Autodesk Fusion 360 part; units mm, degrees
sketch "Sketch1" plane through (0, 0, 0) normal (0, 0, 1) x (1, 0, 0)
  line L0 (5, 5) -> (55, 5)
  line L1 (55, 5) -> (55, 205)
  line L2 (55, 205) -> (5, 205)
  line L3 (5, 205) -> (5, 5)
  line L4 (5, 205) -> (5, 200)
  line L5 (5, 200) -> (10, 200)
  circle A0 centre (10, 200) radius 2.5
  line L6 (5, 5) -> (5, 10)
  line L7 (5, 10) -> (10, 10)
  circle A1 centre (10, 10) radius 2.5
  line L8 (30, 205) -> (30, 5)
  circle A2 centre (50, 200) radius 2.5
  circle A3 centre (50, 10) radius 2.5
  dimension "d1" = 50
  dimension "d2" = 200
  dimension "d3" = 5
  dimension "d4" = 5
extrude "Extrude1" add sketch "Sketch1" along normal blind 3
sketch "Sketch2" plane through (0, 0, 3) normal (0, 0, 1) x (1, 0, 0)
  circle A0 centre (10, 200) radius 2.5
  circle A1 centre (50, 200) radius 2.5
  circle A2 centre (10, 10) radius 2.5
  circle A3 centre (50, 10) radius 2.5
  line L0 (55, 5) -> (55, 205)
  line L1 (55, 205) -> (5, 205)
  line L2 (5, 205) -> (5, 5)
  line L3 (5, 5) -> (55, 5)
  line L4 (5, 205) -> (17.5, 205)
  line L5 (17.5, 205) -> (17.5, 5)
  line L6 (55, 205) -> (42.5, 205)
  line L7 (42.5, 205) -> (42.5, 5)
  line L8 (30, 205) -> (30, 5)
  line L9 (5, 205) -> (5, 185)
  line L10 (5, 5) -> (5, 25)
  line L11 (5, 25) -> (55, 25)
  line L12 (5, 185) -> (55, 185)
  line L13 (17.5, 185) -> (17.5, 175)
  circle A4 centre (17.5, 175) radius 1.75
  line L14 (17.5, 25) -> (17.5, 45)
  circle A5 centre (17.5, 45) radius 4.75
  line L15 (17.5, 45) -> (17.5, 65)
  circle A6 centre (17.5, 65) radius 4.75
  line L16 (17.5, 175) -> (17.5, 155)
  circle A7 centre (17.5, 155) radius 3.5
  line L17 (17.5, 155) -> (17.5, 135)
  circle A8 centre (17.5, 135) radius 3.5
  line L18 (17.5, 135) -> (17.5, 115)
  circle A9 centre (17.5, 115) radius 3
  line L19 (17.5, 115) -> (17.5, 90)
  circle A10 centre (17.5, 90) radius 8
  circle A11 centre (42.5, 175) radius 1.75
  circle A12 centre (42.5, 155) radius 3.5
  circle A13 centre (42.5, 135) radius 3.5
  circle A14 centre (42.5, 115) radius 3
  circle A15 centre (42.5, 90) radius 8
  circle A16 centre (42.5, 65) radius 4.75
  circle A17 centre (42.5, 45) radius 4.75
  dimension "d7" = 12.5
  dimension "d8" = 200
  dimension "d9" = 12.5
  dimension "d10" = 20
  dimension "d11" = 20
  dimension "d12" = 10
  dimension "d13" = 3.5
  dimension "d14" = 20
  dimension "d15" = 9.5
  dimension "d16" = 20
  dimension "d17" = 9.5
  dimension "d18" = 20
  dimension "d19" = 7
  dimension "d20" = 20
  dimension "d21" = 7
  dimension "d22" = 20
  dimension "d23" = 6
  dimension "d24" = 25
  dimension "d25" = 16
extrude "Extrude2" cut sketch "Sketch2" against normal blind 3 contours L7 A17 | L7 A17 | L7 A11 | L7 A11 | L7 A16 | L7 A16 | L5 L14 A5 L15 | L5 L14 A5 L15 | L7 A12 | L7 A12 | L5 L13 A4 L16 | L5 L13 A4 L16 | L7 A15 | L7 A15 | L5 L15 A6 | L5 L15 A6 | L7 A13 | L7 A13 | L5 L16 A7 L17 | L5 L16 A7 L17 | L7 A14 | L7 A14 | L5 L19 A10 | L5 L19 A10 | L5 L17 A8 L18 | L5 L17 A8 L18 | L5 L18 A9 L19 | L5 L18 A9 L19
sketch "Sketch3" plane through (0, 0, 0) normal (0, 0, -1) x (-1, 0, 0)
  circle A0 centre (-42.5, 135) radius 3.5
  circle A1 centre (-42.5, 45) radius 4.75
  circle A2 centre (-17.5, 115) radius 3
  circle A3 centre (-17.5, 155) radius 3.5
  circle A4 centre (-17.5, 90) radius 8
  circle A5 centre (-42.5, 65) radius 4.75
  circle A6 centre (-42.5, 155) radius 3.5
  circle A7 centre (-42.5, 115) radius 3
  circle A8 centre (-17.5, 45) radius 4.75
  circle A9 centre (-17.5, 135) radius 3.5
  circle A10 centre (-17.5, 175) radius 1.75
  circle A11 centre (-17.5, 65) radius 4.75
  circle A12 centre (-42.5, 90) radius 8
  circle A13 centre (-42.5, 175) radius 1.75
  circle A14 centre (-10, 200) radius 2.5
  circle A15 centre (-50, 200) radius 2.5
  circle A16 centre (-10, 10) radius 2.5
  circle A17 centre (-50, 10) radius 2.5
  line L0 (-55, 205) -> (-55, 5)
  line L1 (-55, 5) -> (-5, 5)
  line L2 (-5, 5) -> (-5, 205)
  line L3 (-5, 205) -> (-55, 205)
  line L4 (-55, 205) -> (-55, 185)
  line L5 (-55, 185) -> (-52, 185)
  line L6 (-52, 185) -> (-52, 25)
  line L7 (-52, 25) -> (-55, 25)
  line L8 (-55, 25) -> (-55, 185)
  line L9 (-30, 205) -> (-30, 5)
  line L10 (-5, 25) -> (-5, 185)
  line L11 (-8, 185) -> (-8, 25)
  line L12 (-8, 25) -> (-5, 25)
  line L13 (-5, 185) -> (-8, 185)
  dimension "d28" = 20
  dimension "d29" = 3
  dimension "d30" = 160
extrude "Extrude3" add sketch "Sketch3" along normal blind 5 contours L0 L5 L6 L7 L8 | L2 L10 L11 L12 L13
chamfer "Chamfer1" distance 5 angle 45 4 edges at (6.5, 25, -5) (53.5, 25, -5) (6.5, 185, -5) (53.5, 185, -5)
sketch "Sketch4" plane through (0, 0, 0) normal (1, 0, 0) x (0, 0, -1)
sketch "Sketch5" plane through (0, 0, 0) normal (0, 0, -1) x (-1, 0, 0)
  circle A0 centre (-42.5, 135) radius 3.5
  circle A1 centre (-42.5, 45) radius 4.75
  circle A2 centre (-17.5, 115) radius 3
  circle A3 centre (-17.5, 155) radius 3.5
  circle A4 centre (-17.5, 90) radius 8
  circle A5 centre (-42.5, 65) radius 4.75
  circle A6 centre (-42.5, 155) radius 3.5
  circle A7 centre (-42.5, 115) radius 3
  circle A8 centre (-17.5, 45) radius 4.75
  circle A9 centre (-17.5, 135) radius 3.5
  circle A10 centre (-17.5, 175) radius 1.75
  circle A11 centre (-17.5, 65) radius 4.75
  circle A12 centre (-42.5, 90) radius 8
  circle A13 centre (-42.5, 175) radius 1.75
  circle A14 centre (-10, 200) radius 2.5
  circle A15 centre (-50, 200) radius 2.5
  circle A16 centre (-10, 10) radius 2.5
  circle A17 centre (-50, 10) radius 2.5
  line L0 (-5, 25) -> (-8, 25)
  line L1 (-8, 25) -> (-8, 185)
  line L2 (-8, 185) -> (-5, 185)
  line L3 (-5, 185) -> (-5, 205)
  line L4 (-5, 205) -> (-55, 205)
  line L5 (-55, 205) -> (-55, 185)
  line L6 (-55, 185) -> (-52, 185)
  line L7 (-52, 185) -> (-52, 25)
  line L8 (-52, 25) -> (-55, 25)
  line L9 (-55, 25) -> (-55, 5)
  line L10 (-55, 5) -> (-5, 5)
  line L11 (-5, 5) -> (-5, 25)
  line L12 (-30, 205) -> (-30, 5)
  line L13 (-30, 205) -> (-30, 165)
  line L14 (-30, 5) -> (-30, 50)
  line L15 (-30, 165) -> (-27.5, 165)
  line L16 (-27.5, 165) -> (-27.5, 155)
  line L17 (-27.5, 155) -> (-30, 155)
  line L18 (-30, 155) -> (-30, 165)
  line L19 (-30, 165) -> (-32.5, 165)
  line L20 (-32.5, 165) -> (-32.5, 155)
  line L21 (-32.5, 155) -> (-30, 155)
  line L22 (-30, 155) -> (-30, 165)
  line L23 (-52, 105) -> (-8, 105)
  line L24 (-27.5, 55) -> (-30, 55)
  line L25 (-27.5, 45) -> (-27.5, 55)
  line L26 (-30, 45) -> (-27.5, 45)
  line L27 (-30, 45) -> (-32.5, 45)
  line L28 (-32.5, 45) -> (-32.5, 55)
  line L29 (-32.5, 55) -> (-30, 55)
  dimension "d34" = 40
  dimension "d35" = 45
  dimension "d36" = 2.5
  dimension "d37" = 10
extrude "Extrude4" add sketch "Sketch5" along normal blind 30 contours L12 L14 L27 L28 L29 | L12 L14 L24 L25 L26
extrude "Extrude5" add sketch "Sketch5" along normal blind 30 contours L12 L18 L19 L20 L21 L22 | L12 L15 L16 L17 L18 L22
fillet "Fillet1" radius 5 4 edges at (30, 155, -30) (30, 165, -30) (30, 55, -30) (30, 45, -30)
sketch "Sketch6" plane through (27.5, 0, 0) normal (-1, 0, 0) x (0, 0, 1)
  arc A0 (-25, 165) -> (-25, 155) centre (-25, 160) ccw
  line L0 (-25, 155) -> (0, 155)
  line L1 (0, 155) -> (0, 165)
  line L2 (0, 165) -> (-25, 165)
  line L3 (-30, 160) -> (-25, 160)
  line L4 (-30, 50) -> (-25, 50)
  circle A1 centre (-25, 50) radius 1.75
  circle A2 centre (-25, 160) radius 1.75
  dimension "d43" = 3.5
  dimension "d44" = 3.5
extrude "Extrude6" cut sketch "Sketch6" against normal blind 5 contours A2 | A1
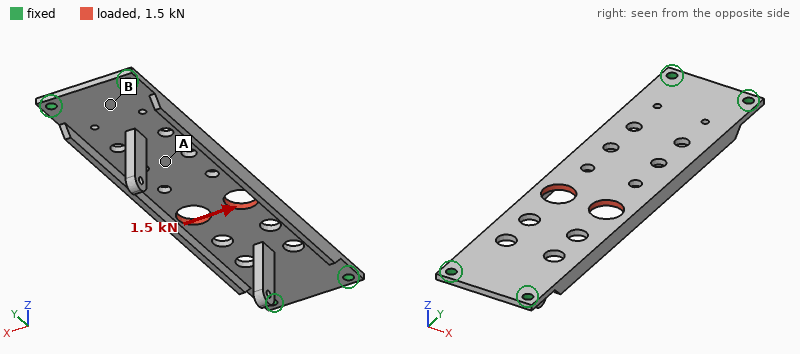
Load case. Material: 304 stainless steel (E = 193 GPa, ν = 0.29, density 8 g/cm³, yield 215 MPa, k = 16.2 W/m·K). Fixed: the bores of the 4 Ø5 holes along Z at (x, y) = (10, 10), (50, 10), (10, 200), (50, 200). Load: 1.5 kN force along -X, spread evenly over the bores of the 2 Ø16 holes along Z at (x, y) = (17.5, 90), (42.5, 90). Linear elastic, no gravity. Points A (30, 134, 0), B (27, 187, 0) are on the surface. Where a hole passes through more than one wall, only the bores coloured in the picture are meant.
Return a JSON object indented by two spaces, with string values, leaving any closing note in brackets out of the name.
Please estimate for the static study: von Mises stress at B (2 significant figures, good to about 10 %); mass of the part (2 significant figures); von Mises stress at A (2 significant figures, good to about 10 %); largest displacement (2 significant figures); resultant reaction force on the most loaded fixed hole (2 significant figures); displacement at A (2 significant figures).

{
  "von Mises stress at B": "7.6 MPa",
  "mass of the part": "280 g",
  "von Mises stress at A": "17 MPa",
  "largest displacement": "28 µm",
  "resultant reaction force on the most loaded fixed hole": "990 N",
  "displacement at A": "12 µm"
}
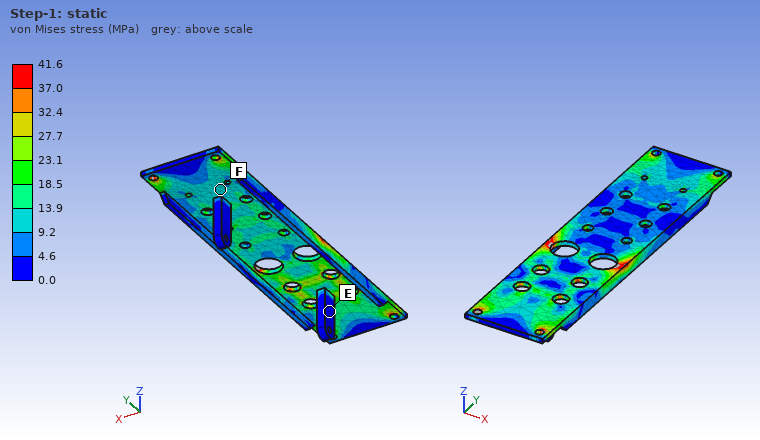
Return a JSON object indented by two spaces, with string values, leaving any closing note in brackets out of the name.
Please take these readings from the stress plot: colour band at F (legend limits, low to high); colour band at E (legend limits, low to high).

{
  "colour band at F": "9.2 to 13.9 MPa",
  "colour band at E": "0.0 to 4.6 MPa"
}
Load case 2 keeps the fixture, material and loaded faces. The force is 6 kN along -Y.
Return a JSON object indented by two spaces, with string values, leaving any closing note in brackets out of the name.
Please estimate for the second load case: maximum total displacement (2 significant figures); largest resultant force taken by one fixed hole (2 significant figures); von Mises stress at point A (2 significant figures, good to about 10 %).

{
  "maximum total displacement": "23 µm",
  "largest resultant force taken by one fixed hole": "1.7 kN",
  "von Mises stress at point A": "14 MPa"
}
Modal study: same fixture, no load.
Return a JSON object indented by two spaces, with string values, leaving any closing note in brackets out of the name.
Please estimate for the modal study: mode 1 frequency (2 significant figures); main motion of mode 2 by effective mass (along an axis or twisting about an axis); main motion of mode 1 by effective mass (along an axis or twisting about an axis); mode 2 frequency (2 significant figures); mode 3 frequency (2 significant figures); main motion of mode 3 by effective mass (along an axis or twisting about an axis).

{
  "mode 1 frequency": "590 Hz",
  "main motion of mode 2 by effective mass": "twisting about Y",
  "main motion of mode 1 by effective mass": "along Z",
  "mode 2 frequency": "1100 Hz",
  "mode 3 frequency": "1700 Hz",
  "main motion of mode 3 by effective mass": "twisting about X"
}
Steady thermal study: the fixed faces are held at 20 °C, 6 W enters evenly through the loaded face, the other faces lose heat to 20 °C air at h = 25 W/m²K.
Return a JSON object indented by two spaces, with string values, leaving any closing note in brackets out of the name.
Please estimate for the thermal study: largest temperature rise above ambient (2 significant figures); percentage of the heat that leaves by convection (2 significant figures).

{
  "largest temperature rise above ambient": "37 K",
  "percentage of the heat that leaves by convection": "93 %"
}
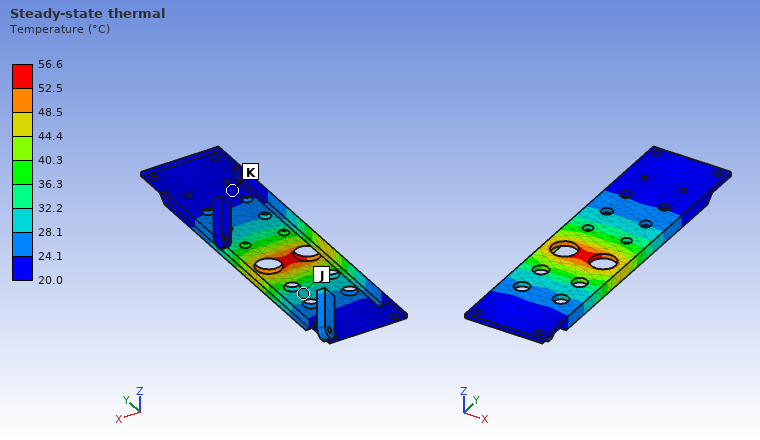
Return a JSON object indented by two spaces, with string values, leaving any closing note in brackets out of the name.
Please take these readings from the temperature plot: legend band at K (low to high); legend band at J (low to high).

{
  "legend band at K": "20.0 to 24.1 °C",
  "legend band at J": "28.1 to 32.2 °C"
}
